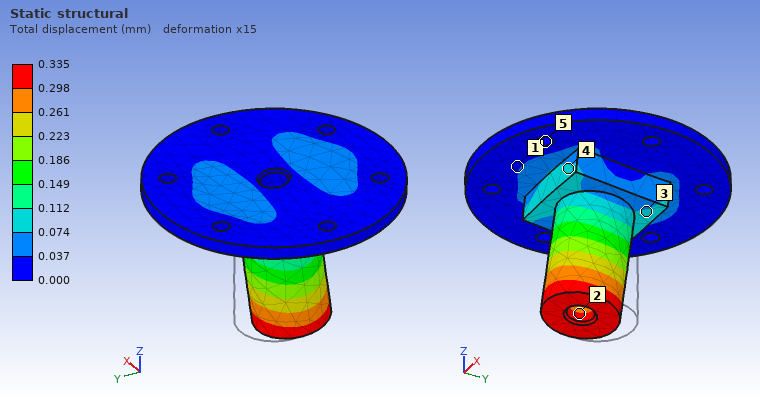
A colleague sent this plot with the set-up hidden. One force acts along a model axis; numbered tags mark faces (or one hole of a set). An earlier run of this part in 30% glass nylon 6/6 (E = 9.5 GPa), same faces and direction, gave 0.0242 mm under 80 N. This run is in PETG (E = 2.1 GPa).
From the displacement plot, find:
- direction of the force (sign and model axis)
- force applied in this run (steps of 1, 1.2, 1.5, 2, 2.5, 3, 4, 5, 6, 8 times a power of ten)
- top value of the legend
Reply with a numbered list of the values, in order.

1. -Y
2. 250 N
3. 0.335 mm
